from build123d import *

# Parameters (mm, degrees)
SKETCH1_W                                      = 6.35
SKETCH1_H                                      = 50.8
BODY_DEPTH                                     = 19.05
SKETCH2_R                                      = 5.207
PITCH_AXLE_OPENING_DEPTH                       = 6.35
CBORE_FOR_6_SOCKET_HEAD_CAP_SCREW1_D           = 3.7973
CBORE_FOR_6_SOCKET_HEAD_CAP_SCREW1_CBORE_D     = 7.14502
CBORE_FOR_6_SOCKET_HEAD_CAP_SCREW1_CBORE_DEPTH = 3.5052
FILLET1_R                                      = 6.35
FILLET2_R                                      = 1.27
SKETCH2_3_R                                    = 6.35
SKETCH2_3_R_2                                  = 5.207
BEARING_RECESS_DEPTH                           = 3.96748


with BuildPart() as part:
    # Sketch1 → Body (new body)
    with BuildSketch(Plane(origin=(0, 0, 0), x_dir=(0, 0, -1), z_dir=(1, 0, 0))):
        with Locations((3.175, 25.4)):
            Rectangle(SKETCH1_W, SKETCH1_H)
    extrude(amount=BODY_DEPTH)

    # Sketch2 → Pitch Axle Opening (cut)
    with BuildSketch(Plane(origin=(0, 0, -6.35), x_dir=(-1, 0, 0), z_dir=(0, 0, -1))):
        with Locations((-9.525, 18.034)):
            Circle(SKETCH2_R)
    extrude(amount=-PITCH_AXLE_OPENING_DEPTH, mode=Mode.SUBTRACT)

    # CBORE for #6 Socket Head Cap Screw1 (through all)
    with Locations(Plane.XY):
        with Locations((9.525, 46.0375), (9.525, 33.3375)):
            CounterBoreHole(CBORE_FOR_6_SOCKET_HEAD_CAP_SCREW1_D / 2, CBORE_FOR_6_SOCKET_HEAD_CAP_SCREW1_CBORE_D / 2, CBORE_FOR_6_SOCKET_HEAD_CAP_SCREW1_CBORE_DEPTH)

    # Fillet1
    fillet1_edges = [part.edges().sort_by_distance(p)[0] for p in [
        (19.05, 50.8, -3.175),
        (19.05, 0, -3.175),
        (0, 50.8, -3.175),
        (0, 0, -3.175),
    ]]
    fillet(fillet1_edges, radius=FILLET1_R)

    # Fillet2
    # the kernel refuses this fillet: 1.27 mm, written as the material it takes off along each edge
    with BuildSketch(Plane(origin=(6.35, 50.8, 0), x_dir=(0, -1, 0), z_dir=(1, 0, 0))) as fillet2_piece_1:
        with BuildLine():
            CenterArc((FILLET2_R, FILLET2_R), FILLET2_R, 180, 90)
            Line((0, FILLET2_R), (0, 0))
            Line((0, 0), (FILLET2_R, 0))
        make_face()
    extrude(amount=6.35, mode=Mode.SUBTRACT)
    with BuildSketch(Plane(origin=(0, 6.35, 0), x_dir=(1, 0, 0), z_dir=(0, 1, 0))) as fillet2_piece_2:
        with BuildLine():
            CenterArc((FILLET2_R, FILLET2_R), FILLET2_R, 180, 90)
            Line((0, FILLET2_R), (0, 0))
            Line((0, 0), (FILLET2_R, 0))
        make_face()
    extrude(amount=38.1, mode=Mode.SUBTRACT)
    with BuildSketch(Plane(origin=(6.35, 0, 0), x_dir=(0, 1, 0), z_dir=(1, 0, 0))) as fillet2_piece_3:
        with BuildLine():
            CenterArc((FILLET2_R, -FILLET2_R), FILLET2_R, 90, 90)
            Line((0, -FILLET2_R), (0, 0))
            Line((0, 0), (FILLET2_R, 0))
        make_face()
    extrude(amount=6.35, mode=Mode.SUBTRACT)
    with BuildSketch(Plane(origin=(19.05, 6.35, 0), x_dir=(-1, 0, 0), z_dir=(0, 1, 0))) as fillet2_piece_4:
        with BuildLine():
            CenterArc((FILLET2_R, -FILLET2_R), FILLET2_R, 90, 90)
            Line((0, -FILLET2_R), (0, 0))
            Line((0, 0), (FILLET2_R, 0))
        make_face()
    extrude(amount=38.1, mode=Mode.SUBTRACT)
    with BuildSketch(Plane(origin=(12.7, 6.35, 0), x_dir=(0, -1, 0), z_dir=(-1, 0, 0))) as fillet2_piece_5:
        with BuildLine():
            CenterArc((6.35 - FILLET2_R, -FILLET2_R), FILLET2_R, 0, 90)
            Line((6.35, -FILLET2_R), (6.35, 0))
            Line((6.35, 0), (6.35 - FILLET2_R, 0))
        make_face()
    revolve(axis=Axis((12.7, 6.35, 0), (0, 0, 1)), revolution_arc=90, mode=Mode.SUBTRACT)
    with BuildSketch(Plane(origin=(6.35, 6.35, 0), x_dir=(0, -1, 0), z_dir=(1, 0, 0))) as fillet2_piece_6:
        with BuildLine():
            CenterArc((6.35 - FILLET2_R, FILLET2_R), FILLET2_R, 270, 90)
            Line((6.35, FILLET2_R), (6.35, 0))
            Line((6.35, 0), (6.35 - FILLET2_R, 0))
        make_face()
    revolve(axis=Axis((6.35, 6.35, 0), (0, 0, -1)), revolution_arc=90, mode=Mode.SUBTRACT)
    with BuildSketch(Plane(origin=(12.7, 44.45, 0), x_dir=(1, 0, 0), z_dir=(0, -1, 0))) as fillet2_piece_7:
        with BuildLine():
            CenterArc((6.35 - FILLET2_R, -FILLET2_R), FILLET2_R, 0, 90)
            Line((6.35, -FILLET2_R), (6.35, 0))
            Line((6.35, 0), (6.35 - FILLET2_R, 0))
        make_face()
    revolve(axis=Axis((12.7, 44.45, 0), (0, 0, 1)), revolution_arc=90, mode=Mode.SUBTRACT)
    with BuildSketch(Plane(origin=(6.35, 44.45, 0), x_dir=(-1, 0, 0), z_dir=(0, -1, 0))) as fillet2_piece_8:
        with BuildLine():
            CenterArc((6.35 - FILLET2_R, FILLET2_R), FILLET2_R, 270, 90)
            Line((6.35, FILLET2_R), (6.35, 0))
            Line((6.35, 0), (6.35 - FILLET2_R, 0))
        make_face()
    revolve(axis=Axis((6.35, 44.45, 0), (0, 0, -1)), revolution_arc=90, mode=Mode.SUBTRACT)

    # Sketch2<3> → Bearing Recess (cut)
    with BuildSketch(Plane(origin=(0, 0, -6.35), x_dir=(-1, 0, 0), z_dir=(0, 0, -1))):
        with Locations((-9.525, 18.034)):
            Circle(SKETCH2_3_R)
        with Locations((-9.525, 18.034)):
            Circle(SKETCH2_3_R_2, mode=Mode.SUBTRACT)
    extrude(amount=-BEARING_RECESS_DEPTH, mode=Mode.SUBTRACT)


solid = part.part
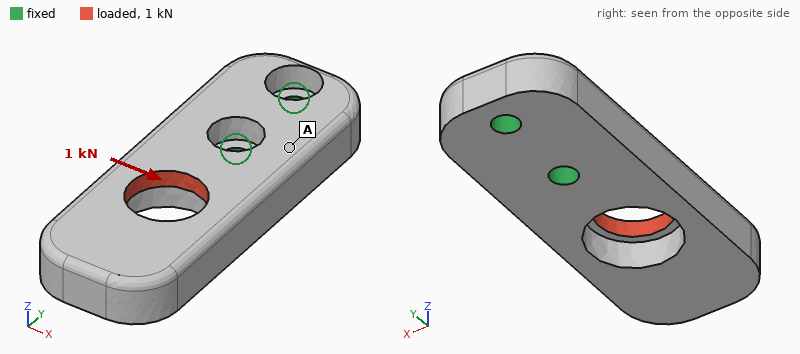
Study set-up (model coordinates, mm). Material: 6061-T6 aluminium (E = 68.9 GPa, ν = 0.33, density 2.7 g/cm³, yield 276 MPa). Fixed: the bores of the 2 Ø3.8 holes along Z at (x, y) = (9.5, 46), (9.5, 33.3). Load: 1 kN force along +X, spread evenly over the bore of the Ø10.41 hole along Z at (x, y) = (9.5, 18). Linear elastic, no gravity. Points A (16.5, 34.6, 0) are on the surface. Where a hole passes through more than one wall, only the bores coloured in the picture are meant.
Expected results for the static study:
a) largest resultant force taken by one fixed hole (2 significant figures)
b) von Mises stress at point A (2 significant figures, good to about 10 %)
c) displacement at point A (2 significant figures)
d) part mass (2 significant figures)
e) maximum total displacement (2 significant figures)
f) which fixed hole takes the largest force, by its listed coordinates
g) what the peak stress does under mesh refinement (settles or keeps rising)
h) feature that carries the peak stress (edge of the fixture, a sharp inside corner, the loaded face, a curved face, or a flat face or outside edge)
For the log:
1.8 kN
24 MPa
12 µm
13 g
75 µm
(9.5, 33.3)
keeps rising
edge of the fixture
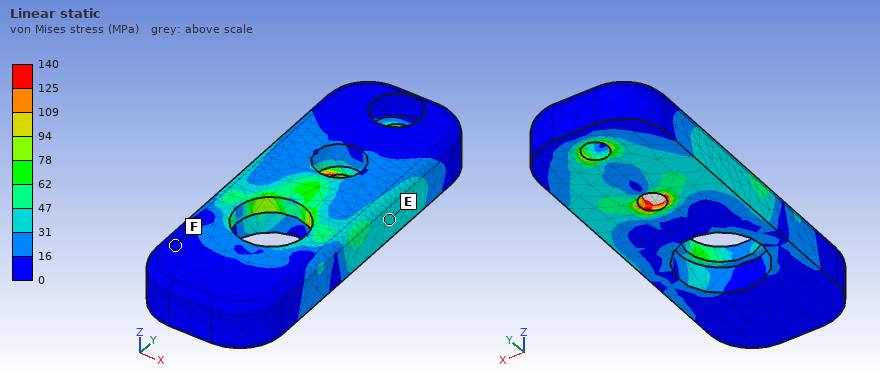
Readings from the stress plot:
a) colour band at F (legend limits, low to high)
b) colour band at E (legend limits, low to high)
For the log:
0 to 16 MPa
31 to 47 MPa
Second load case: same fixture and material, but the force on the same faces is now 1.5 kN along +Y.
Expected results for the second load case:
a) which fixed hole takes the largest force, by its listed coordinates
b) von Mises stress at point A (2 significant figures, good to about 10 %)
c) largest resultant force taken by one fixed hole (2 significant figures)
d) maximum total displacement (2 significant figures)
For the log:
(9.5, 33.3)
36 MPa
910 N
90 µm
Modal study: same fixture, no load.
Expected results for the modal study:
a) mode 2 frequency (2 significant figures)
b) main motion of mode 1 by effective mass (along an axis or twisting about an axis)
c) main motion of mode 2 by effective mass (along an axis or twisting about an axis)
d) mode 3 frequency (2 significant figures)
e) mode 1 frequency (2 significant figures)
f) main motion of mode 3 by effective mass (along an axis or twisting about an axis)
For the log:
7200 Hz
along Z
along X
9400 Hz
3500 Hz
twisting about Y
